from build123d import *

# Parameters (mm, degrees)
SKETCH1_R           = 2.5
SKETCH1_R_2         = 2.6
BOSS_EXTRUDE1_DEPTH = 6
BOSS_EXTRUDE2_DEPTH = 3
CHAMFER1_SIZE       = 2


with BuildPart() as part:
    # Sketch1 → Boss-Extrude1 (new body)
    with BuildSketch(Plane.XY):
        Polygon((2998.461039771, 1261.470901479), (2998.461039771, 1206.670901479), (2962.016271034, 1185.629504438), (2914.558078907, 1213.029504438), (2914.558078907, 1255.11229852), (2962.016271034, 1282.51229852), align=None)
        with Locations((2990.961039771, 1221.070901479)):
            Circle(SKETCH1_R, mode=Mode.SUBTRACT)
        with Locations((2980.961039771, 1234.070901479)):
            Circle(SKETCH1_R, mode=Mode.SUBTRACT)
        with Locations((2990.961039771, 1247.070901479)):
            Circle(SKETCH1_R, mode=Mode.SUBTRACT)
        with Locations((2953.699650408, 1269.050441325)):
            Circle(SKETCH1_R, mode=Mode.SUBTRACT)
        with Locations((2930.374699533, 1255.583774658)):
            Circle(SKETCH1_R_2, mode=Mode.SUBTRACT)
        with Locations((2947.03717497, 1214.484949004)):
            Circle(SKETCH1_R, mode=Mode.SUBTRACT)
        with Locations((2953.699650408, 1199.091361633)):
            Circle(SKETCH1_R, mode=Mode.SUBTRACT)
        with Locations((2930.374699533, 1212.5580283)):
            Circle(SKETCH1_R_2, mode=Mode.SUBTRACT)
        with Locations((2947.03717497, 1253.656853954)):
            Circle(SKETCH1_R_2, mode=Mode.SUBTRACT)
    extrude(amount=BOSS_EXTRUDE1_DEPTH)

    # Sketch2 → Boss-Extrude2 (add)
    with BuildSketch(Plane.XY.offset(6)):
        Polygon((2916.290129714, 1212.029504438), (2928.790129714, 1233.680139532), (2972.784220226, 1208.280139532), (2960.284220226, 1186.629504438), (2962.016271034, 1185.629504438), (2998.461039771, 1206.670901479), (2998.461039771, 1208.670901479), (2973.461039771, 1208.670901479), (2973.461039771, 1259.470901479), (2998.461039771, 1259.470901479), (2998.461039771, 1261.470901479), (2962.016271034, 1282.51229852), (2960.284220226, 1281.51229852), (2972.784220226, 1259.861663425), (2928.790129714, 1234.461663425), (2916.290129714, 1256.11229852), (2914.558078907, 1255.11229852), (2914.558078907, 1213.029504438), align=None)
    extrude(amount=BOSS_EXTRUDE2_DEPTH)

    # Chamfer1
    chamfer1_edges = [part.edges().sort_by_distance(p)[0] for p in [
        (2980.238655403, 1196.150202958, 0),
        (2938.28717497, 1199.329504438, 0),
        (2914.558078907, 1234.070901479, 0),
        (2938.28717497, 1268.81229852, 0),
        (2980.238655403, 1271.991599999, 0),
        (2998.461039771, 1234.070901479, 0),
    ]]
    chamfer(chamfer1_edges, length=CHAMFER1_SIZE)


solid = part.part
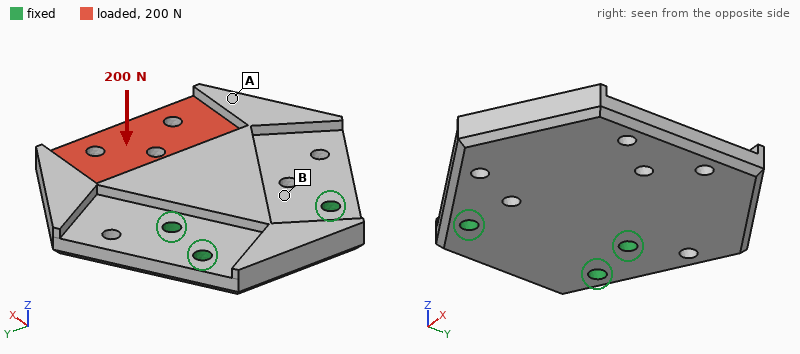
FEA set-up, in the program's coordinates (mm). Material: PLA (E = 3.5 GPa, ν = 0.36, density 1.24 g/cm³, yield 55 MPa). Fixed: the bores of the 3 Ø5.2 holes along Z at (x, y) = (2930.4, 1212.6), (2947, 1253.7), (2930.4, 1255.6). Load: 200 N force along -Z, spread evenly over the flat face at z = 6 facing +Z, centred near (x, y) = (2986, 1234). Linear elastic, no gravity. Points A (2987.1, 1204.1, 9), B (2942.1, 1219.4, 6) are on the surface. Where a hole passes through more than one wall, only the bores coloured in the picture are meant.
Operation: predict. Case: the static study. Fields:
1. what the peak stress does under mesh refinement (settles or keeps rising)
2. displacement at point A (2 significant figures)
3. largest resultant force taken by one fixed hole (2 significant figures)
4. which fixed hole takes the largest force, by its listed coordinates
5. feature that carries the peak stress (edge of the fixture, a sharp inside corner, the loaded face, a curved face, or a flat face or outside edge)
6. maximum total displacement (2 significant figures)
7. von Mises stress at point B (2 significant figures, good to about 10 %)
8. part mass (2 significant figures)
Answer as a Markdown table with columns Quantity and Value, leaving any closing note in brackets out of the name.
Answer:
| Quantity | Value |
|---|---|
| what the peak stress does under mesh refinement | keeps rising |
| displacement at point A | 1.2 mm |
| largest resultant force taken by one fixed hole | 340 N |
| which fixed hole takes the largest force, by its listed coordinates | (2947, 1253.7) |
| feature that carries the peak stress | edge of the fixture |
| maximum total displacement | 1.5 mm |
| von Mises stress at point B | 6.6 MPa |
| part mass | 51 g |
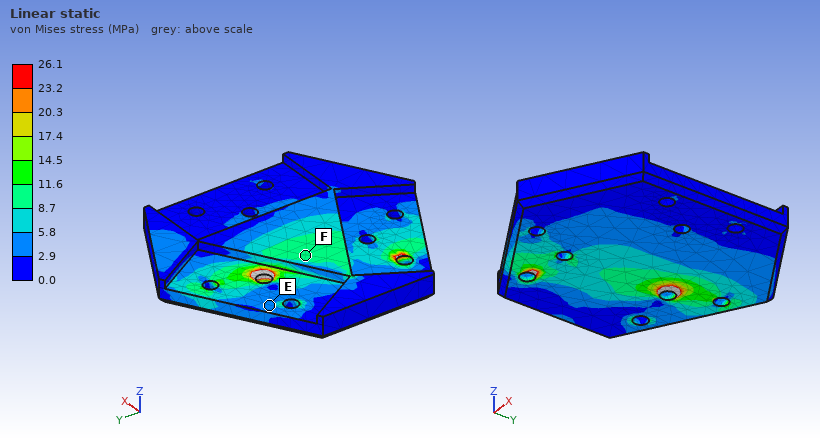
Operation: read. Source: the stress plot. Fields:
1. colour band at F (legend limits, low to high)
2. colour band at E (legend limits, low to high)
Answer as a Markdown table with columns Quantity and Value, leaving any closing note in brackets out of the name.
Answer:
| Quantity | Value |
|---|---|
| colour band at F | 8.7 to 11.6 MPa |
| colour band at E | 2.9 to 5.8 MPa |
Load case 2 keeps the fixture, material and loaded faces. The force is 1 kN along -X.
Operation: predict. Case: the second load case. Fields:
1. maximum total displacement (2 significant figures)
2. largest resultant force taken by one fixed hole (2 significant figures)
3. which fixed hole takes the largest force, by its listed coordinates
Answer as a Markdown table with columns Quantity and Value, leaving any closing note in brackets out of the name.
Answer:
| Quantity | Value |
|---|---|
| maximum total displacement | 0.60 mm |
| largest resultant force taken by one fixed hole | 460 N |
| which fixed hole takes the largest force, by its listed coordinates | (2930.4, 1212.6) |
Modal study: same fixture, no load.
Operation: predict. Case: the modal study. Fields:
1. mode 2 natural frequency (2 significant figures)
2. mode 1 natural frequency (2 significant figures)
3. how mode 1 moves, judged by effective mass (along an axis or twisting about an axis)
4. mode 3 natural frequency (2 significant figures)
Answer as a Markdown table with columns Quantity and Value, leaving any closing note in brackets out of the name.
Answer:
| Quantity | Value |
|---|---|
| mode 2 natural frequency | 1000 Hz |
| mode 1 natural frequency | 540 Hz |
| how mode 1 moves, judged by effective mass | along Z |
| mode 3 natural frequency | 2000 Hz |
